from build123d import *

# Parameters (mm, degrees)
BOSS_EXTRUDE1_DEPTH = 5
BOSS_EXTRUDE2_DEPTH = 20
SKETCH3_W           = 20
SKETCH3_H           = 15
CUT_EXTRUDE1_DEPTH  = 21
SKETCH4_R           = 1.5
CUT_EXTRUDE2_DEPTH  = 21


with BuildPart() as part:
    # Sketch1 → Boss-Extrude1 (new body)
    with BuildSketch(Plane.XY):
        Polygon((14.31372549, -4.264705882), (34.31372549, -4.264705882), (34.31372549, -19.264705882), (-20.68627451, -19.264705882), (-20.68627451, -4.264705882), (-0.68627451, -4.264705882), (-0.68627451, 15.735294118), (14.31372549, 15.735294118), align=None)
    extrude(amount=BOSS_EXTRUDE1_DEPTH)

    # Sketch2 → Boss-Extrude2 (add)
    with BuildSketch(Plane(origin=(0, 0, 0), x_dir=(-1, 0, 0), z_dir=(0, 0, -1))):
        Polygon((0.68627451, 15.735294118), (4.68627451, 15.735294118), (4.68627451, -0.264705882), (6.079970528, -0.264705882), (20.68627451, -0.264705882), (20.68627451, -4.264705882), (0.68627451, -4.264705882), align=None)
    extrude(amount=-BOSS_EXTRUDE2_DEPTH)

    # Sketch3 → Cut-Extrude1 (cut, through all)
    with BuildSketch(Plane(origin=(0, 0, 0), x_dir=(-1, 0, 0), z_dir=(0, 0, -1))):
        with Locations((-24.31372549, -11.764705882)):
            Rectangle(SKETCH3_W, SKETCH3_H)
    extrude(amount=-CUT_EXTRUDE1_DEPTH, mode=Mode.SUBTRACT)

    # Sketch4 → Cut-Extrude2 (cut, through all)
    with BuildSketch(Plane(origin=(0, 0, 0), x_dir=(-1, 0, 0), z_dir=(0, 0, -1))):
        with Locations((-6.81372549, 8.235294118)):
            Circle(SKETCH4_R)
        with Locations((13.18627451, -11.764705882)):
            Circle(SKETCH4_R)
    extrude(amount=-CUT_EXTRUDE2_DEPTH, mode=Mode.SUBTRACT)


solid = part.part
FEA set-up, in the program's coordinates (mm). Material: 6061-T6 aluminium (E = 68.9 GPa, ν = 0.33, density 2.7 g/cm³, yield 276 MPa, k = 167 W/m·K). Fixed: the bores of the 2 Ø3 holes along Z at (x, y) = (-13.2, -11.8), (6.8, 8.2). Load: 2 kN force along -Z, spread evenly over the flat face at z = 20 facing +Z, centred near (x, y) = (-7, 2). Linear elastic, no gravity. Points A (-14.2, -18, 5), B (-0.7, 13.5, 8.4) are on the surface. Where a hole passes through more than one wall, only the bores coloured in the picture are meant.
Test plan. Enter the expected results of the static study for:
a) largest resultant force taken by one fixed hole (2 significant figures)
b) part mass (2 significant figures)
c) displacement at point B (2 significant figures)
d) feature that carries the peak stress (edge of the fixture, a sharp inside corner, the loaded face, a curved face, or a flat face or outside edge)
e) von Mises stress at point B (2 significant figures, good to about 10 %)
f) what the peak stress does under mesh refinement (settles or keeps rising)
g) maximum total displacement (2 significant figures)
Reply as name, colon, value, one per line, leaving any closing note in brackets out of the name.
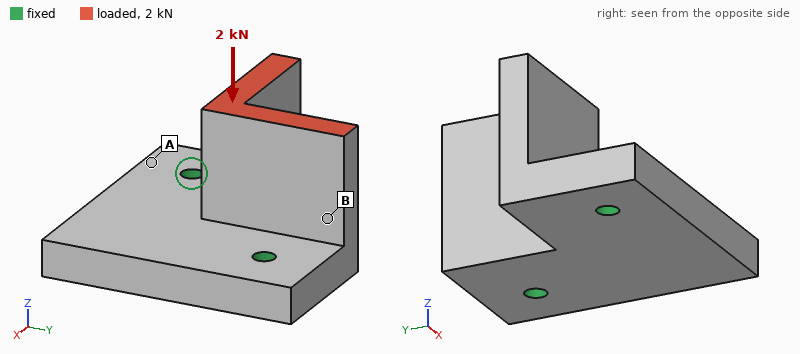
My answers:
largest resultant force taken by one fixed hole: 1.0 kN
part mass: 19 g
displacement at point B: 31 µm
feature that carries the peak stress: edge of the fixture
von Mises stress at point B: 39 MPa
what the peak stress does under mesh refinement: keeps rising
maximum total displacement: 55 µm
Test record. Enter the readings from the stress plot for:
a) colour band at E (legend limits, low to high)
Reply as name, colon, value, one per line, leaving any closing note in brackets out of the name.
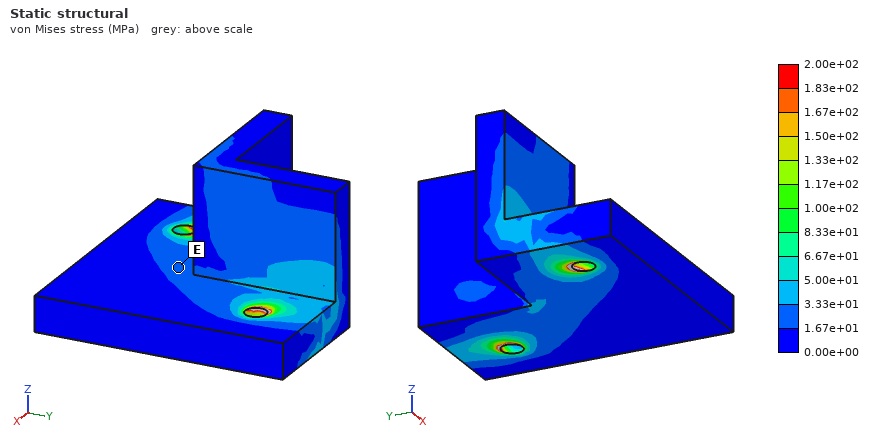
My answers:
colour band at E: 1.67e+01 to 3.33e+01 MPa
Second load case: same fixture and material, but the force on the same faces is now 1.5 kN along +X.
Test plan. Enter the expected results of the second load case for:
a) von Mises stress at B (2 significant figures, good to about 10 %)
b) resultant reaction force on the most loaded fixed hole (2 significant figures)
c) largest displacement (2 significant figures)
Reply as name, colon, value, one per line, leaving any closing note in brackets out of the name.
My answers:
von Mises stress at B: 78 MPa
resultant reaction force on the most loaded fixed hole: 1.1 kN
largest displacement: 0.17 mm
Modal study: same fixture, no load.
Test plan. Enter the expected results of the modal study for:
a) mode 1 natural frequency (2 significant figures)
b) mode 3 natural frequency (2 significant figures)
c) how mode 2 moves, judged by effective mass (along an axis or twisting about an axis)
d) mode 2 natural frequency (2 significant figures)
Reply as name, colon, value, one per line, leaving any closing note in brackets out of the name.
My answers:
mode 1 natural frequency: 7900 Hz
mode 3 natural frequency: 14 kHz
how mode 2 moves, judged by effective mass: along Z
mode 2 natural frequency: 12 kHz
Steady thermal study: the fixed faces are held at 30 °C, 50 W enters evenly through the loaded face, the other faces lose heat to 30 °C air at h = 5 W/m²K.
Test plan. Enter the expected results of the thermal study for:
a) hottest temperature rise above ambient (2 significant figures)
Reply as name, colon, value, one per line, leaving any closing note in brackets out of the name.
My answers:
hottest temperature rise above ambient: 50 K
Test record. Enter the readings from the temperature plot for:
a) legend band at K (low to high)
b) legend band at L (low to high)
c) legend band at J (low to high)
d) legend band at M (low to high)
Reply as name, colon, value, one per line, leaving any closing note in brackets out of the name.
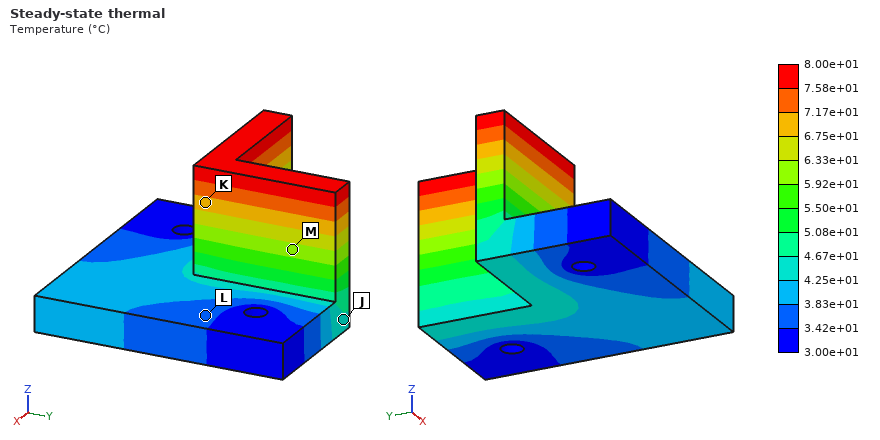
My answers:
legend band at K: 6.75e+01 to 7.17e+01 °C
legend band at L: 3.42e+01 to 3.83e+01 °C
legend band at J: 4.25e+01 to 4.67e+01 °C
legend band at M: 5.92e+01 to 6.33e+01 °C
